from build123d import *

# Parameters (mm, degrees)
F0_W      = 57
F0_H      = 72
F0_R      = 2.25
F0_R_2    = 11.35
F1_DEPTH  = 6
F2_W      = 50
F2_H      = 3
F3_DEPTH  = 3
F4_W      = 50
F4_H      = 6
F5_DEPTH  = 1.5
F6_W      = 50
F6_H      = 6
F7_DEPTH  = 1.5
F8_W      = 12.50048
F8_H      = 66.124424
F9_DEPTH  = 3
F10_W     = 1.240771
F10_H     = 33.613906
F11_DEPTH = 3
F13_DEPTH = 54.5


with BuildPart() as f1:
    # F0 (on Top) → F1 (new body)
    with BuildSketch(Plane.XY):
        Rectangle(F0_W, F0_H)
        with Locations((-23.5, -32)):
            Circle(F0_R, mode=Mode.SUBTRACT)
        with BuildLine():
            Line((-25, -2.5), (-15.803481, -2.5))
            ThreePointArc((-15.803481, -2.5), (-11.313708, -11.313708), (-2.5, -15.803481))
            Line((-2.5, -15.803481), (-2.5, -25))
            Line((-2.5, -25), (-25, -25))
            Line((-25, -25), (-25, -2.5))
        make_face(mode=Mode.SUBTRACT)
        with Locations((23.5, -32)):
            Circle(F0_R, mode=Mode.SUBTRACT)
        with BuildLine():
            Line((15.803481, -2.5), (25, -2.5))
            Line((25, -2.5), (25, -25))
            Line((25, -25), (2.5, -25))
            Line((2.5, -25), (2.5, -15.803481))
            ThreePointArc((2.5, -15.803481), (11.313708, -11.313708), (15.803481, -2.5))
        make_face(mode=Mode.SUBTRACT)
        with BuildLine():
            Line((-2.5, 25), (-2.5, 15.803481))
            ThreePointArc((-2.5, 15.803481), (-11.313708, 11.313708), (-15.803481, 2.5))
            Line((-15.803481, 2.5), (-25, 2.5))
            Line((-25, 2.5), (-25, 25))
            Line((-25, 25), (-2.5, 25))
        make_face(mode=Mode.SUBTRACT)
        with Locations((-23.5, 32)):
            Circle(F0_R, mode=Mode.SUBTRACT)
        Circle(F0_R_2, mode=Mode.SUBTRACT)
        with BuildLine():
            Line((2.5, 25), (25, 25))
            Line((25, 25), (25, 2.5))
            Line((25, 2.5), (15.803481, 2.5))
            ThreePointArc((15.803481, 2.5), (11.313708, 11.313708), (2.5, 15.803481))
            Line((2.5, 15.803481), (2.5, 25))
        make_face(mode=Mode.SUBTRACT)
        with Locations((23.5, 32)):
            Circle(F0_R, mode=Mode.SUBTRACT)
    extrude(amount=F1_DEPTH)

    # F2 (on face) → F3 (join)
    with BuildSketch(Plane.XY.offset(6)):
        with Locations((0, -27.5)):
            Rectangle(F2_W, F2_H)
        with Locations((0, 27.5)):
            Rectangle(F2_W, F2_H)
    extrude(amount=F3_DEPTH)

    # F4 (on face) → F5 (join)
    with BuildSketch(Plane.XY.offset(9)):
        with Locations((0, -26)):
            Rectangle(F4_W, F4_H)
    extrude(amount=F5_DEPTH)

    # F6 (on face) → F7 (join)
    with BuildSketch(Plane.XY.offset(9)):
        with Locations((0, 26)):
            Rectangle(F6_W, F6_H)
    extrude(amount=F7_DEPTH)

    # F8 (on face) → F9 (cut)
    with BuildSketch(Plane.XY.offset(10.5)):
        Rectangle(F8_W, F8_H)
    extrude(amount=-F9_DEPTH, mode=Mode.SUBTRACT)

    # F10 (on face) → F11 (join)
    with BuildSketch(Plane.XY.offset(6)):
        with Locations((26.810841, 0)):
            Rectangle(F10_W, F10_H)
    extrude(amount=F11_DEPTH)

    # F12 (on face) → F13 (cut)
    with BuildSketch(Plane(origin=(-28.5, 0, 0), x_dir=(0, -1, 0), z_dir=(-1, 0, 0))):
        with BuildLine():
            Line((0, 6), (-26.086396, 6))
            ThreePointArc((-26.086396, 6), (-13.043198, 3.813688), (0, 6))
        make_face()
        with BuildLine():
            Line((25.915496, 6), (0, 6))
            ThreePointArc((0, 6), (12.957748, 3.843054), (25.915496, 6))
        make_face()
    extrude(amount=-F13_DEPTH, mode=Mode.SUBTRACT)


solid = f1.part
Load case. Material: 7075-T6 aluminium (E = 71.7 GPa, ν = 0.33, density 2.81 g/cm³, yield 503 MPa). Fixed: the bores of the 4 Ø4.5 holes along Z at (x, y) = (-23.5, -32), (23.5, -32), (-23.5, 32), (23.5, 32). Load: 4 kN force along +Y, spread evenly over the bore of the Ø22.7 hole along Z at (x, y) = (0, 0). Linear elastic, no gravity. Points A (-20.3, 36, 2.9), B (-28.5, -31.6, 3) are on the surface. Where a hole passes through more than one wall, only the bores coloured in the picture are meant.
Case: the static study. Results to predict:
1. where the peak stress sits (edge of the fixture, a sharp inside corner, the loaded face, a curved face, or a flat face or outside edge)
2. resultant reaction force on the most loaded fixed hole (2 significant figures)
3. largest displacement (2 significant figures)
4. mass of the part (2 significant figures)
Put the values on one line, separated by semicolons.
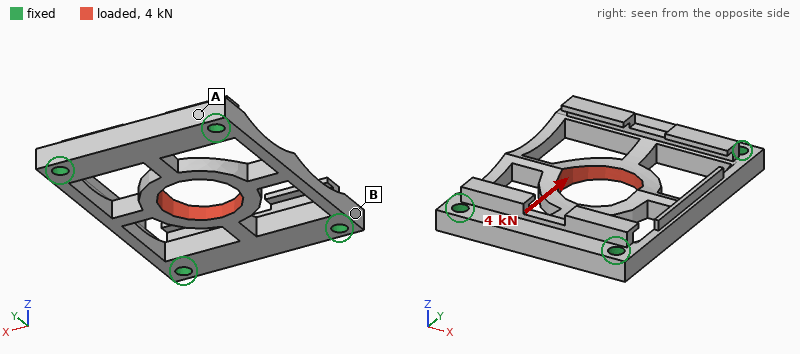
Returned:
the loaded face; 1.1 kN; 86 µm; 37 g
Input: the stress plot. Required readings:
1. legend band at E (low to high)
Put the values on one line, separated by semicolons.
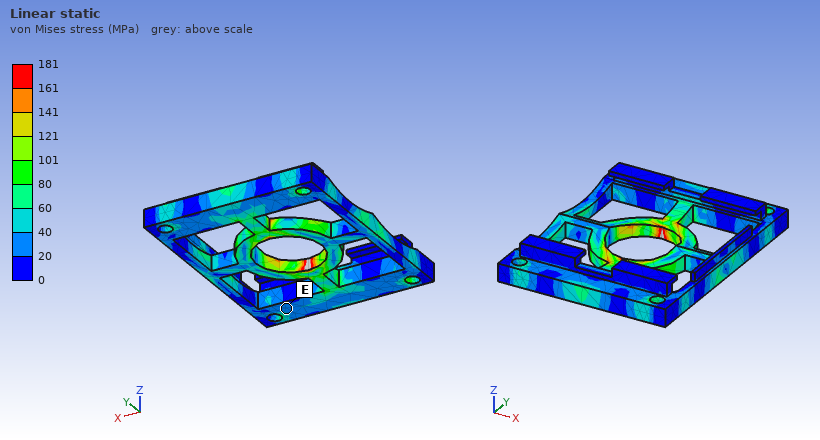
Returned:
20 to 40 MPa
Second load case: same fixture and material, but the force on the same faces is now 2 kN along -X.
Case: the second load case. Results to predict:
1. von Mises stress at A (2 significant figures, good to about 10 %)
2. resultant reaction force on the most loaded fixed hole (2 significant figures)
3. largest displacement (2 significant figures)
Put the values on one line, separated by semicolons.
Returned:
12 MPa; 570 N; 79 µm
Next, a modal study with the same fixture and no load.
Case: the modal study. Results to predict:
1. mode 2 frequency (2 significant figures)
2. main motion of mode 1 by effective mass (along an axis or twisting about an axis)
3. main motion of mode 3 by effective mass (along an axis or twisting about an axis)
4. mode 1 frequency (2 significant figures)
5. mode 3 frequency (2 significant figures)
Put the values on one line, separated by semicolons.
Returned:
6800 Hz; along Z; along X; 5400 Hz; 8800 Hz
